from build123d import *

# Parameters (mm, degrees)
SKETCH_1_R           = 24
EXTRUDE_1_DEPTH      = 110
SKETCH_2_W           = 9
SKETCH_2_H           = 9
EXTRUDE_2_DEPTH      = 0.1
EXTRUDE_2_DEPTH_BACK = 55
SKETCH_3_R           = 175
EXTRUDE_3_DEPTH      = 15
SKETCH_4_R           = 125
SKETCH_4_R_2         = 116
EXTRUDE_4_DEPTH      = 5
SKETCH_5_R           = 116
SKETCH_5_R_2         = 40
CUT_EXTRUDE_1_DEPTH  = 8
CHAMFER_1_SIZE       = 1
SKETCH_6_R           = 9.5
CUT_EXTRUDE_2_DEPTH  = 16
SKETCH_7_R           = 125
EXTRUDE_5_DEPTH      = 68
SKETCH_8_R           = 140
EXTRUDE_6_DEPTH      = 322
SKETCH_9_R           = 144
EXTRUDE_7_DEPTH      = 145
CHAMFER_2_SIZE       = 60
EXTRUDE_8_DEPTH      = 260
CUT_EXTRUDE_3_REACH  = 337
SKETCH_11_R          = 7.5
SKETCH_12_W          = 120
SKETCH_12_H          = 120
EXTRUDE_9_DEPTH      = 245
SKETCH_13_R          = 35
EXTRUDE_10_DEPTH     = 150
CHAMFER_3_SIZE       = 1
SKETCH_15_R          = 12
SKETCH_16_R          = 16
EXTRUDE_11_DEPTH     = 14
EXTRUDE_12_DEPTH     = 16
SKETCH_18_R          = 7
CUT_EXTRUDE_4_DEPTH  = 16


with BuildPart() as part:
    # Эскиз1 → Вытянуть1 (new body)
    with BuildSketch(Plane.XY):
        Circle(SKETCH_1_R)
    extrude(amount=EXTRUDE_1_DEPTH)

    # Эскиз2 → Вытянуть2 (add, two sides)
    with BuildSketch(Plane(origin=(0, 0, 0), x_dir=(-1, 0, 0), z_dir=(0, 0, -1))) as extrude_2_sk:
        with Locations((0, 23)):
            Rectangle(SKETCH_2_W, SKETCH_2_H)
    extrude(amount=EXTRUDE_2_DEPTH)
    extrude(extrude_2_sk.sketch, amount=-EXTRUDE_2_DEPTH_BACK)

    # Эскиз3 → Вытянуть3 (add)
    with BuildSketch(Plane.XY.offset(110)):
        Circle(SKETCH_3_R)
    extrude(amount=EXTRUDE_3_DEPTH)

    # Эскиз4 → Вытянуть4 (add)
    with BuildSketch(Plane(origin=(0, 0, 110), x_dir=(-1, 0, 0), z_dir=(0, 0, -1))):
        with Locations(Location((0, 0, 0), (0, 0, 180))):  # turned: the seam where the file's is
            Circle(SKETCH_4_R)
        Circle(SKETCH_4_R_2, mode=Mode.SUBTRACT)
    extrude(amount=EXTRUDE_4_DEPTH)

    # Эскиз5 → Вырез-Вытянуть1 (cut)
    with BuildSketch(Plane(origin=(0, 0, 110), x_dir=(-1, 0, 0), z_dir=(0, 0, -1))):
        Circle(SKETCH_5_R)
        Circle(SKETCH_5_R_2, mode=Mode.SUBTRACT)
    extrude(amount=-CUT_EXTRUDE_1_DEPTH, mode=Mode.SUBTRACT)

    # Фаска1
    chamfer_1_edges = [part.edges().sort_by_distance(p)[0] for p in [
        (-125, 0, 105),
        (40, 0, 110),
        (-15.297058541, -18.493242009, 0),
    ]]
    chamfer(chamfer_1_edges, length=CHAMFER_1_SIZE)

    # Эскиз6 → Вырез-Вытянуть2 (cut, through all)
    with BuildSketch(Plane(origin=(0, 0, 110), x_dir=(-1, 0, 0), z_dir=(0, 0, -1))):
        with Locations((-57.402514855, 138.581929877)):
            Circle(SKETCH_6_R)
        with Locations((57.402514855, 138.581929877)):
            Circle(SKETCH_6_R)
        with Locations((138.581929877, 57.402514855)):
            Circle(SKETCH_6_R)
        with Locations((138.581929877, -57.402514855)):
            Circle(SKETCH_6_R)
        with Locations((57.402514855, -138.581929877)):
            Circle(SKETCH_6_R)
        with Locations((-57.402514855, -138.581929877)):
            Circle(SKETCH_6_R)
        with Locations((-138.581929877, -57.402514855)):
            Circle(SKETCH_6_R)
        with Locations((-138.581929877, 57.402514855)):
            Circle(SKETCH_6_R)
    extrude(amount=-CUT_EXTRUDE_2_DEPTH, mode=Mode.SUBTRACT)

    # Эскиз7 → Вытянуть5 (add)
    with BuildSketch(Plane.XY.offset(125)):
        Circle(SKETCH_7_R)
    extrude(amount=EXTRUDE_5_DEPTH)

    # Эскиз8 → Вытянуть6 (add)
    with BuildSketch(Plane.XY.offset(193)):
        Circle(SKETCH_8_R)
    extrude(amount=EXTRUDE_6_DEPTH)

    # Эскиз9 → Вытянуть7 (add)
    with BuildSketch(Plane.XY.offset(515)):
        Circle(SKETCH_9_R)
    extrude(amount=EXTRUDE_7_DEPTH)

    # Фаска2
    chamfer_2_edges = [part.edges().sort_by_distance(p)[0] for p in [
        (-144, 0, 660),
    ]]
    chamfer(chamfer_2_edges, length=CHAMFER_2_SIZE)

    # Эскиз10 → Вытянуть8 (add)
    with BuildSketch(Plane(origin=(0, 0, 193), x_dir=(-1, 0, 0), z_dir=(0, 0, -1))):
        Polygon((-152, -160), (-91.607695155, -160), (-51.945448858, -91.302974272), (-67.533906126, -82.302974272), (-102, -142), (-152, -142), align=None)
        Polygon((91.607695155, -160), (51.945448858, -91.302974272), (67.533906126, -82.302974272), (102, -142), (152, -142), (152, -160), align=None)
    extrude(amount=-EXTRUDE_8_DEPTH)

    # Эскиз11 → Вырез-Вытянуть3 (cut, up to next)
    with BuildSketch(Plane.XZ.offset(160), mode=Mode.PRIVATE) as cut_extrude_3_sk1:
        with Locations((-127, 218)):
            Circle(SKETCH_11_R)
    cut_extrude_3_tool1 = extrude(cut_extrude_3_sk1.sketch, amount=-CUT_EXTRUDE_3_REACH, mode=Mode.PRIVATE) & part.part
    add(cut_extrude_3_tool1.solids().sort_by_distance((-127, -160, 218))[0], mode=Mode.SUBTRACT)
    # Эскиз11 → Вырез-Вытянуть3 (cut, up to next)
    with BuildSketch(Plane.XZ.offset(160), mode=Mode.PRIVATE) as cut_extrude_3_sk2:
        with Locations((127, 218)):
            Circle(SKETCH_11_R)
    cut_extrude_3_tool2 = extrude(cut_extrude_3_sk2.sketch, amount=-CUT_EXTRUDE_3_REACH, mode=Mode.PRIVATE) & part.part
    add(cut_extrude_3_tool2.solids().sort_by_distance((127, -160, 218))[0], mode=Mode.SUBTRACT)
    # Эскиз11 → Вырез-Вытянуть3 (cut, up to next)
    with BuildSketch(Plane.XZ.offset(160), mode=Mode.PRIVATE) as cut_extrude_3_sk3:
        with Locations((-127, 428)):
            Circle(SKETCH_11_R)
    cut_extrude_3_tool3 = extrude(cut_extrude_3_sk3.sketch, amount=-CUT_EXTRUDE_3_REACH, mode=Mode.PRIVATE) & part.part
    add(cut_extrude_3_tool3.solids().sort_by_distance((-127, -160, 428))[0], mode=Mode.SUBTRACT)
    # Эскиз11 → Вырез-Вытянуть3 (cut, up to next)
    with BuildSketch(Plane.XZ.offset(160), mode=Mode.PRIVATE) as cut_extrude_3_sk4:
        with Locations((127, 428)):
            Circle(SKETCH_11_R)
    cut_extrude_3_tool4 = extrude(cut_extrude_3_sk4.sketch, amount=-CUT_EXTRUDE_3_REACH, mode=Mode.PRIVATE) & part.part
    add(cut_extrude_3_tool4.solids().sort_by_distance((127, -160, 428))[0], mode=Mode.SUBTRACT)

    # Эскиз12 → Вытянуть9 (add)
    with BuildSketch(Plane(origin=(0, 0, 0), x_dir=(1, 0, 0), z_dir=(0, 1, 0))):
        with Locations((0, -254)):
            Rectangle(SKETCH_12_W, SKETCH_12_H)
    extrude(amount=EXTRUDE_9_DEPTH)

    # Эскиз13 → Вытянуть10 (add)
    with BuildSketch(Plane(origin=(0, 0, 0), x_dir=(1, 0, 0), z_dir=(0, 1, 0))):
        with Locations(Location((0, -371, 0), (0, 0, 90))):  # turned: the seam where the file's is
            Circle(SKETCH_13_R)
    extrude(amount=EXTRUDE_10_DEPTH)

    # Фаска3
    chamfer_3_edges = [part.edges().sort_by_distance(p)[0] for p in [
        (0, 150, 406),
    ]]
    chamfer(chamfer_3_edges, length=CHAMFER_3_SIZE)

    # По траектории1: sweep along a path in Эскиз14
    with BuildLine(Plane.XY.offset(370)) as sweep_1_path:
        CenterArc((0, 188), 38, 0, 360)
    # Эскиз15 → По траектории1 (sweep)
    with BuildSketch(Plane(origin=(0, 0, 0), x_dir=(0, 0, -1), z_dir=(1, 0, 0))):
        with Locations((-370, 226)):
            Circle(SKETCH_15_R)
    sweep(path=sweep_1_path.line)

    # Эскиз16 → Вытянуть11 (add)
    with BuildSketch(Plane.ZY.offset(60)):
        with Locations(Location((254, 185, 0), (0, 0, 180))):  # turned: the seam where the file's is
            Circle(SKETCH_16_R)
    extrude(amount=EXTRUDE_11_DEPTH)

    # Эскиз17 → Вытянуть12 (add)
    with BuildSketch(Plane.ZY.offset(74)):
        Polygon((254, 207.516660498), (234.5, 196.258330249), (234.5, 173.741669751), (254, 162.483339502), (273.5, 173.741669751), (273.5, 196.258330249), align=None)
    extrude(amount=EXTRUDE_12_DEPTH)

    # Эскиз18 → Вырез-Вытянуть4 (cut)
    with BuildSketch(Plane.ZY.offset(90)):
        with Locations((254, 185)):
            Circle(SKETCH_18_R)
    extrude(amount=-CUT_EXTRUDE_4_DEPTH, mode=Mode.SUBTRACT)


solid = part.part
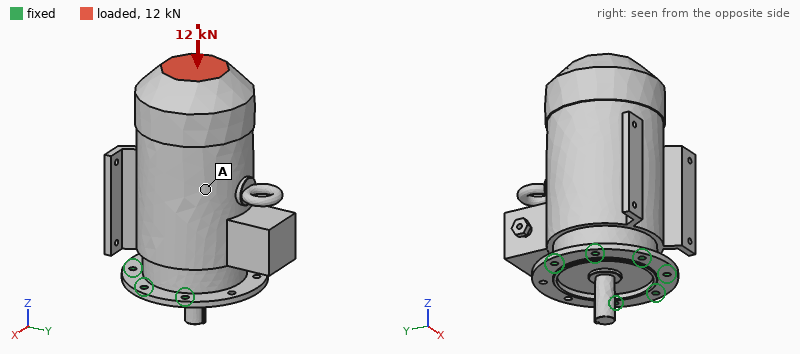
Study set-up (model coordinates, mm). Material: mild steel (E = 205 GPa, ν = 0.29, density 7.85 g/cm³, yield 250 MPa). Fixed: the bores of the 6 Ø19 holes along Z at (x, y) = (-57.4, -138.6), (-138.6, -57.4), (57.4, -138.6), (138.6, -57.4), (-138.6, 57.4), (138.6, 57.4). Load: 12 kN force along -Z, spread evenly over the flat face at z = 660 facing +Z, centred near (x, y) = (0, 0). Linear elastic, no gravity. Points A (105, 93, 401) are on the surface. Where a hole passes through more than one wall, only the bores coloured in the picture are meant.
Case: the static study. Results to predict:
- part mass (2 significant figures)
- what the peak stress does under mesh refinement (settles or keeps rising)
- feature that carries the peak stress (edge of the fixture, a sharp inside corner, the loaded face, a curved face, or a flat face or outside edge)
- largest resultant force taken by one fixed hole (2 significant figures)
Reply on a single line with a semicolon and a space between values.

280 kg; keeps rising; edge of the fixture; 4.0 kN
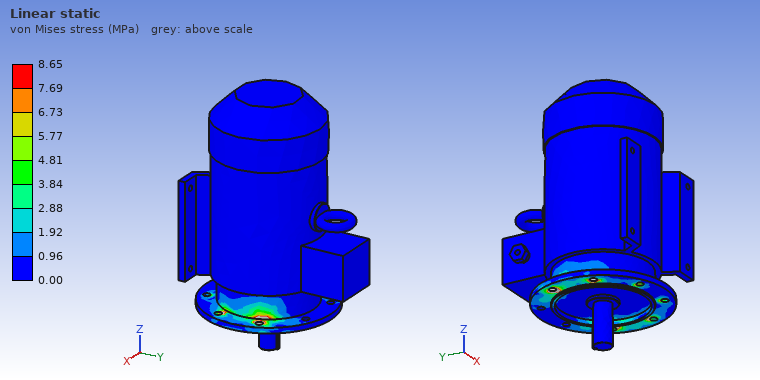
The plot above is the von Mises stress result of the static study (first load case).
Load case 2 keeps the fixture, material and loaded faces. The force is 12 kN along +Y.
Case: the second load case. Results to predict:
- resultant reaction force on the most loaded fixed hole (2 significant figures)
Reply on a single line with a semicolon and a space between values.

22 kN
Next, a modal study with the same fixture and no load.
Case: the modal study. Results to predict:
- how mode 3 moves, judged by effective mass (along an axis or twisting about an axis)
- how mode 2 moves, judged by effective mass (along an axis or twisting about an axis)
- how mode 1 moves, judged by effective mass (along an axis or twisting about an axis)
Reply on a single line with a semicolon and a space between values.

along Z; along X; along Y
